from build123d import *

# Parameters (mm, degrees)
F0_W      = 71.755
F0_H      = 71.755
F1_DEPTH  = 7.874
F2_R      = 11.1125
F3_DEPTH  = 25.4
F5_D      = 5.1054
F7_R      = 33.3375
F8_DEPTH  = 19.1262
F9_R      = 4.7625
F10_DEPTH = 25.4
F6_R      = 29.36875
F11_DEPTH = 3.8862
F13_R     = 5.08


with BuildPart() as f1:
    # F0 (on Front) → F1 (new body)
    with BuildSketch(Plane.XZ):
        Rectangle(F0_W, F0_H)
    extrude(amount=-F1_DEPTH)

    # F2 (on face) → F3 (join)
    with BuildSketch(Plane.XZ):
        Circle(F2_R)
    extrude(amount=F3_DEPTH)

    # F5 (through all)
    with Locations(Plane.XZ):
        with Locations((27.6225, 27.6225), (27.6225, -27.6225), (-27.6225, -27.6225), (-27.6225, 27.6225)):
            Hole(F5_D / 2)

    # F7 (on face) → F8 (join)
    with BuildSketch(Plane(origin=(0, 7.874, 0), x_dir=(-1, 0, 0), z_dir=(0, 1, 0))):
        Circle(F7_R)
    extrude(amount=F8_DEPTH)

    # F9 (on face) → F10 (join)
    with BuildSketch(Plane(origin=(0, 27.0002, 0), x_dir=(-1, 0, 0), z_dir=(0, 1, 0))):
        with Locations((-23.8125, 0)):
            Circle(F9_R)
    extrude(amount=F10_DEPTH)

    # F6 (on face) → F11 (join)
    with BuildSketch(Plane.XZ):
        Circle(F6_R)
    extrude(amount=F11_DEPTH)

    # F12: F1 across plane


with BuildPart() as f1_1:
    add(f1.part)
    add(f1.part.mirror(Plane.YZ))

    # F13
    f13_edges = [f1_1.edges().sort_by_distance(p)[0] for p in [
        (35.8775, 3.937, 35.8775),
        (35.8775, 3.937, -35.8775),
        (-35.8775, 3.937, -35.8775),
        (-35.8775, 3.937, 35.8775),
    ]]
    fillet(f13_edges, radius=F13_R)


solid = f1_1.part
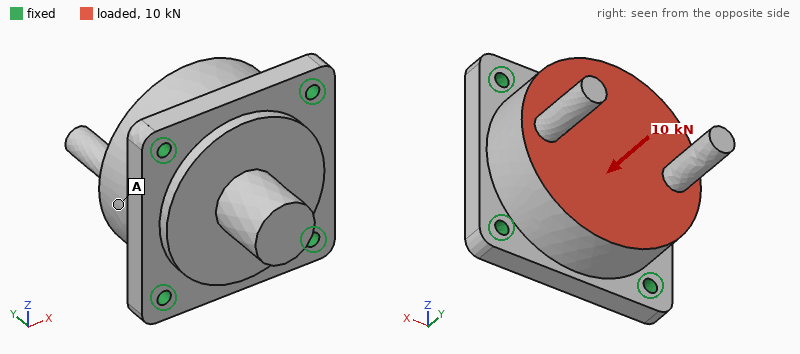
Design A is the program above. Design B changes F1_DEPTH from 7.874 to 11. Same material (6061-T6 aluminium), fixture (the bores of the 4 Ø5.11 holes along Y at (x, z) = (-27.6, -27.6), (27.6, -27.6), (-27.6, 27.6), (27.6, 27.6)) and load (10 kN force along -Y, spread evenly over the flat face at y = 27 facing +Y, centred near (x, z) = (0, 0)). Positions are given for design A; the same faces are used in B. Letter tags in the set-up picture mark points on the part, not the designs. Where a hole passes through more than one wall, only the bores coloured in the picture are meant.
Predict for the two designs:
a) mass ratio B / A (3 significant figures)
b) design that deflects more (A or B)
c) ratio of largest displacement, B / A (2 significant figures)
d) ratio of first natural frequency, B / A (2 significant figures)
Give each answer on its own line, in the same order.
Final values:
1.04
A
0.71
1.0
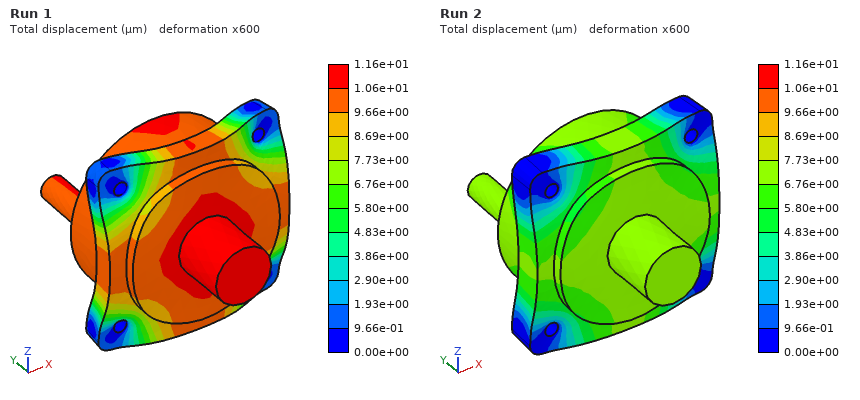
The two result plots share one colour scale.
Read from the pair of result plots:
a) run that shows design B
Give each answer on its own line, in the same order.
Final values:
Run 2
